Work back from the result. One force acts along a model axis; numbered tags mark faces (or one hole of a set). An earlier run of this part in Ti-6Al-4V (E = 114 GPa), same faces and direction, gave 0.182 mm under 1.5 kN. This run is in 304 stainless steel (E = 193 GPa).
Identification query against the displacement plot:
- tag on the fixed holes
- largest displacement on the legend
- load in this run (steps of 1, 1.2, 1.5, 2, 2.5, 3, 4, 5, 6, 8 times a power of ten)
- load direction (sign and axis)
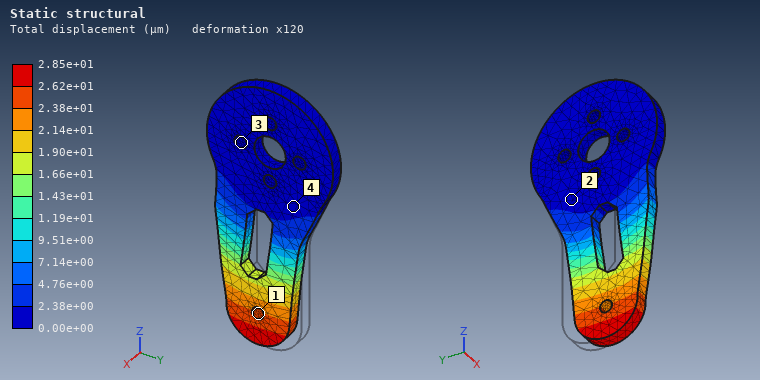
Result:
3
2.85e+01 µm
400 N
-Y
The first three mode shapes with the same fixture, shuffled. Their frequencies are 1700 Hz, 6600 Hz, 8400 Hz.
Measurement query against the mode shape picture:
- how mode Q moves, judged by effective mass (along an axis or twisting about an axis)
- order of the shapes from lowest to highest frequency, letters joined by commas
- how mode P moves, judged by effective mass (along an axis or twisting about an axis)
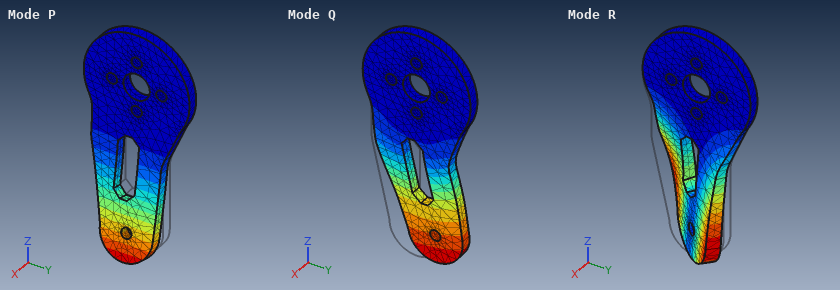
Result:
along Y
P, R, Q
along X
